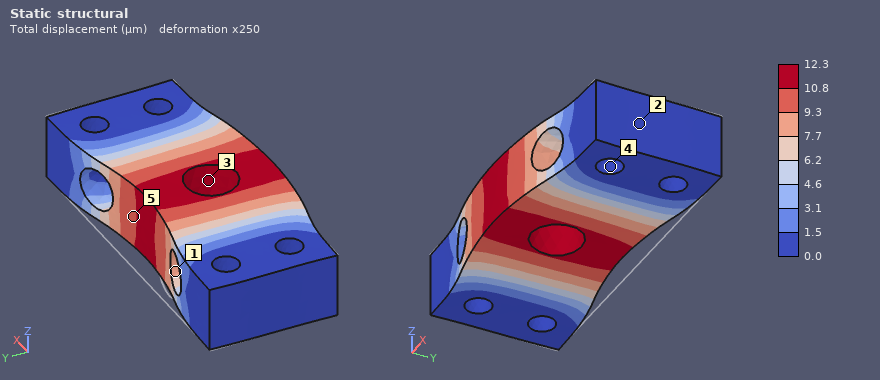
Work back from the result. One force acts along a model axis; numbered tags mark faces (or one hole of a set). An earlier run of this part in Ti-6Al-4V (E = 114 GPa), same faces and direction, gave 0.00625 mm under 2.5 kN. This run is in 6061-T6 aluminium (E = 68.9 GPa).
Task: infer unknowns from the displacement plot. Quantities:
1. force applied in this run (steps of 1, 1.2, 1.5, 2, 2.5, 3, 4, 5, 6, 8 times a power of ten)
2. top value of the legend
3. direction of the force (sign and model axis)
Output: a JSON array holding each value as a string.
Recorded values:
["3 kN", "12.3 µm", "-Y"]
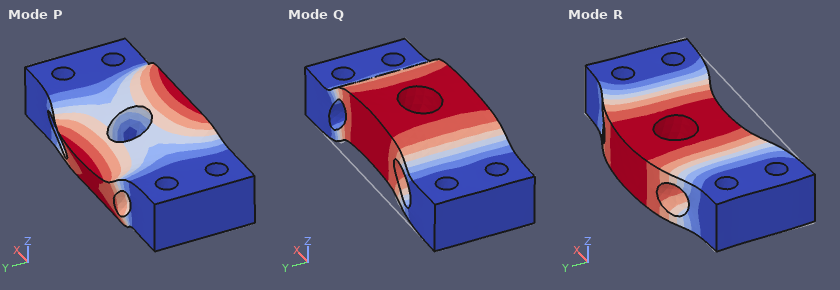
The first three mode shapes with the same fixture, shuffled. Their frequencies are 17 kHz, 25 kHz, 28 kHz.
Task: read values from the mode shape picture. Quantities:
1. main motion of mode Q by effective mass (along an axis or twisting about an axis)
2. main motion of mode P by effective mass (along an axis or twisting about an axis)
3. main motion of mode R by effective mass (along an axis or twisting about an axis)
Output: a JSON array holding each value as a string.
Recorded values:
["along Z", "twisting about X", "along Y"]
